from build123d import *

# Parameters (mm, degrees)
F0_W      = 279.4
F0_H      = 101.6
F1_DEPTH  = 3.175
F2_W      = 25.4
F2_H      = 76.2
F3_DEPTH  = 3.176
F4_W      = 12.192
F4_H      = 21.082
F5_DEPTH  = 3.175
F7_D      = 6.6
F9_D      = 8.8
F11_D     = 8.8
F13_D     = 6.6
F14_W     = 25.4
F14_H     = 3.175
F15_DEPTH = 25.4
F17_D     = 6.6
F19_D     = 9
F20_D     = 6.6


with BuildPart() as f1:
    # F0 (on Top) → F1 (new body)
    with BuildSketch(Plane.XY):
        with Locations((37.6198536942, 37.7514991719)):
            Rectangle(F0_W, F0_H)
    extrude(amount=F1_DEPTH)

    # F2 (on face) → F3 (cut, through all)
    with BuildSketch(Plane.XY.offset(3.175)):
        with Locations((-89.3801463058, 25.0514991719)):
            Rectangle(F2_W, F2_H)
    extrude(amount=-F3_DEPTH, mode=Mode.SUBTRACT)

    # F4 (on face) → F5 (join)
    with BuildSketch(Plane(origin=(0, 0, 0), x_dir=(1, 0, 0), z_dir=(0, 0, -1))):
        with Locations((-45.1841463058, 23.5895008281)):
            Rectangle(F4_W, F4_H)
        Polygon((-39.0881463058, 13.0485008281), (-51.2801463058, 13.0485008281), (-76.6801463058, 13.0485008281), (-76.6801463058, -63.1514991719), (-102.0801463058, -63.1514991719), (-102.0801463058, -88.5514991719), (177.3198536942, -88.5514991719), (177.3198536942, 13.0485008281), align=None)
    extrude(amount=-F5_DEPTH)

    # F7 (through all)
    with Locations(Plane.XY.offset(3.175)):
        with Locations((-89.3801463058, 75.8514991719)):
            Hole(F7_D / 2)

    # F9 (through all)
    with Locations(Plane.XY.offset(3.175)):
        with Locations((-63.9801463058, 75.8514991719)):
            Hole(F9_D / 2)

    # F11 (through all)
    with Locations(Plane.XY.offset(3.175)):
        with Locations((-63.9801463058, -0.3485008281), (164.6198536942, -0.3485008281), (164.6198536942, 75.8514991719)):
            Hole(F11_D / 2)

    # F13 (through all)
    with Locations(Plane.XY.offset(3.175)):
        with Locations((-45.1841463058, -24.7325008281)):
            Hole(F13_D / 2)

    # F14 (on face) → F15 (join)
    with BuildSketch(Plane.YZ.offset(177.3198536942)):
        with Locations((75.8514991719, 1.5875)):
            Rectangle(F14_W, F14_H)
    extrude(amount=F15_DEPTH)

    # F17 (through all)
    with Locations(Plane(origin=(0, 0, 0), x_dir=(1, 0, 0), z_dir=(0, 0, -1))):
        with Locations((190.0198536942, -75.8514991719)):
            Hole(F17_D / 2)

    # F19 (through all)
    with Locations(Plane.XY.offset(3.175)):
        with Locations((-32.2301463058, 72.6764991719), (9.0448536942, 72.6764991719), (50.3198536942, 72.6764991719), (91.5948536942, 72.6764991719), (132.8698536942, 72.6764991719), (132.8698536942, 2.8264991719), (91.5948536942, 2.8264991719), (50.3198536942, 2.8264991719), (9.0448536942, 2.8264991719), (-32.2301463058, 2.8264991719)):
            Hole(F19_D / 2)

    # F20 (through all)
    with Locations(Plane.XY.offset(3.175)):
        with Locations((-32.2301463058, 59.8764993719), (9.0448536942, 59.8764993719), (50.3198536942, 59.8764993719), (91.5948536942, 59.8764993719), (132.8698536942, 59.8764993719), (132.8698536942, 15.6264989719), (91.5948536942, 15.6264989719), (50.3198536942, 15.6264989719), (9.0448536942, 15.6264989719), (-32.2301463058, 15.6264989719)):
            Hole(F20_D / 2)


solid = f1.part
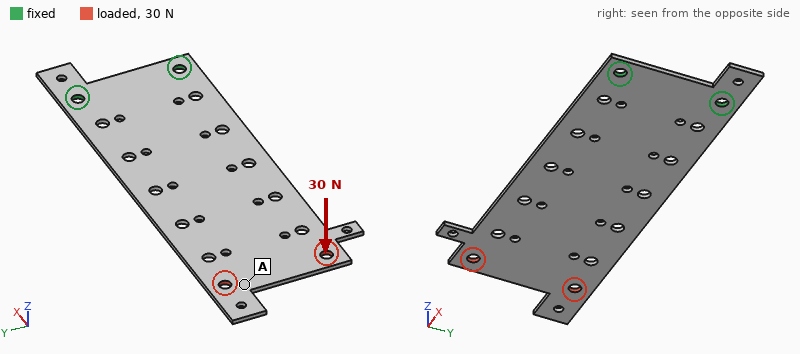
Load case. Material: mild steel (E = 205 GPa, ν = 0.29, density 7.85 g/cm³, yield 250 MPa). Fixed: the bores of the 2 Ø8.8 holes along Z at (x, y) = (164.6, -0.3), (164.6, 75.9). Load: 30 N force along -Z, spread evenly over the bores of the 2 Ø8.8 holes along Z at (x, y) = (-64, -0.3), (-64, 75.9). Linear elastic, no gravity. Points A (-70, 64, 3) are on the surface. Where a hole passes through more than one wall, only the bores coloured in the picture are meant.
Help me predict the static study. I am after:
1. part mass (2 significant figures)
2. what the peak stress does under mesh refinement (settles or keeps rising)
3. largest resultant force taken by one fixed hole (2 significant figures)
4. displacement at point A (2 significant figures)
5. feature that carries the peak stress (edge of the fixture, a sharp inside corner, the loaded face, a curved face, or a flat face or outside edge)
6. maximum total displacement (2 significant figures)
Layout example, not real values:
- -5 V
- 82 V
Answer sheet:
- 650 g
- keeps rising
- 16 N
- 2.5 mm
- edge of the fixture
- 3.0 mm
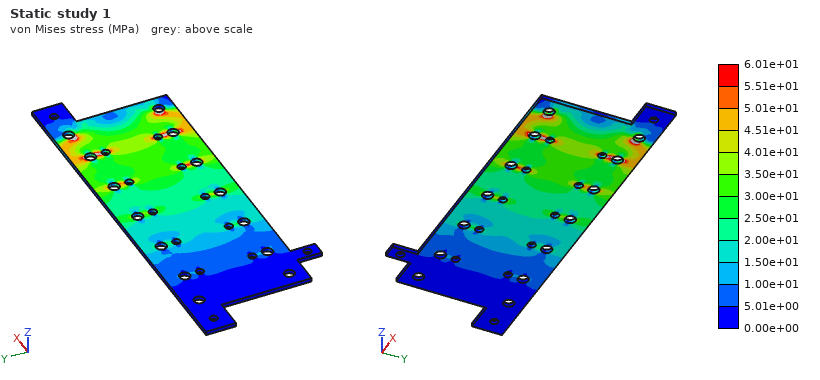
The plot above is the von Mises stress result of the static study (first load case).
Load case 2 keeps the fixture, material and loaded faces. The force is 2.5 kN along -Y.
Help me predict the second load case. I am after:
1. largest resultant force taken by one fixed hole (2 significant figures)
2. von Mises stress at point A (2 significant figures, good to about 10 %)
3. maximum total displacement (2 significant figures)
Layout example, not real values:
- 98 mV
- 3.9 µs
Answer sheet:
- 7.4 kN
- 13 MPa
- 0.30 mm
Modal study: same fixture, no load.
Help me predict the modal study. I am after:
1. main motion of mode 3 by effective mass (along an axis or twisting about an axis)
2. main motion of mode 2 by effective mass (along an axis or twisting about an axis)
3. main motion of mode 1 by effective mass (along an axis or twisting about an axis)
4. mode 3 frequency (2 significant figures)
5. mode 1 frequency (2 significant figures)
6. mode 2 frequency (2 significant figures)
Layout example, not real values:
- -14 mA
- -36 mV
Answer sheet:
- along Z
- twisting about X
- along Z
- 260 Hz
- 41 Hz
- 210 Hz
